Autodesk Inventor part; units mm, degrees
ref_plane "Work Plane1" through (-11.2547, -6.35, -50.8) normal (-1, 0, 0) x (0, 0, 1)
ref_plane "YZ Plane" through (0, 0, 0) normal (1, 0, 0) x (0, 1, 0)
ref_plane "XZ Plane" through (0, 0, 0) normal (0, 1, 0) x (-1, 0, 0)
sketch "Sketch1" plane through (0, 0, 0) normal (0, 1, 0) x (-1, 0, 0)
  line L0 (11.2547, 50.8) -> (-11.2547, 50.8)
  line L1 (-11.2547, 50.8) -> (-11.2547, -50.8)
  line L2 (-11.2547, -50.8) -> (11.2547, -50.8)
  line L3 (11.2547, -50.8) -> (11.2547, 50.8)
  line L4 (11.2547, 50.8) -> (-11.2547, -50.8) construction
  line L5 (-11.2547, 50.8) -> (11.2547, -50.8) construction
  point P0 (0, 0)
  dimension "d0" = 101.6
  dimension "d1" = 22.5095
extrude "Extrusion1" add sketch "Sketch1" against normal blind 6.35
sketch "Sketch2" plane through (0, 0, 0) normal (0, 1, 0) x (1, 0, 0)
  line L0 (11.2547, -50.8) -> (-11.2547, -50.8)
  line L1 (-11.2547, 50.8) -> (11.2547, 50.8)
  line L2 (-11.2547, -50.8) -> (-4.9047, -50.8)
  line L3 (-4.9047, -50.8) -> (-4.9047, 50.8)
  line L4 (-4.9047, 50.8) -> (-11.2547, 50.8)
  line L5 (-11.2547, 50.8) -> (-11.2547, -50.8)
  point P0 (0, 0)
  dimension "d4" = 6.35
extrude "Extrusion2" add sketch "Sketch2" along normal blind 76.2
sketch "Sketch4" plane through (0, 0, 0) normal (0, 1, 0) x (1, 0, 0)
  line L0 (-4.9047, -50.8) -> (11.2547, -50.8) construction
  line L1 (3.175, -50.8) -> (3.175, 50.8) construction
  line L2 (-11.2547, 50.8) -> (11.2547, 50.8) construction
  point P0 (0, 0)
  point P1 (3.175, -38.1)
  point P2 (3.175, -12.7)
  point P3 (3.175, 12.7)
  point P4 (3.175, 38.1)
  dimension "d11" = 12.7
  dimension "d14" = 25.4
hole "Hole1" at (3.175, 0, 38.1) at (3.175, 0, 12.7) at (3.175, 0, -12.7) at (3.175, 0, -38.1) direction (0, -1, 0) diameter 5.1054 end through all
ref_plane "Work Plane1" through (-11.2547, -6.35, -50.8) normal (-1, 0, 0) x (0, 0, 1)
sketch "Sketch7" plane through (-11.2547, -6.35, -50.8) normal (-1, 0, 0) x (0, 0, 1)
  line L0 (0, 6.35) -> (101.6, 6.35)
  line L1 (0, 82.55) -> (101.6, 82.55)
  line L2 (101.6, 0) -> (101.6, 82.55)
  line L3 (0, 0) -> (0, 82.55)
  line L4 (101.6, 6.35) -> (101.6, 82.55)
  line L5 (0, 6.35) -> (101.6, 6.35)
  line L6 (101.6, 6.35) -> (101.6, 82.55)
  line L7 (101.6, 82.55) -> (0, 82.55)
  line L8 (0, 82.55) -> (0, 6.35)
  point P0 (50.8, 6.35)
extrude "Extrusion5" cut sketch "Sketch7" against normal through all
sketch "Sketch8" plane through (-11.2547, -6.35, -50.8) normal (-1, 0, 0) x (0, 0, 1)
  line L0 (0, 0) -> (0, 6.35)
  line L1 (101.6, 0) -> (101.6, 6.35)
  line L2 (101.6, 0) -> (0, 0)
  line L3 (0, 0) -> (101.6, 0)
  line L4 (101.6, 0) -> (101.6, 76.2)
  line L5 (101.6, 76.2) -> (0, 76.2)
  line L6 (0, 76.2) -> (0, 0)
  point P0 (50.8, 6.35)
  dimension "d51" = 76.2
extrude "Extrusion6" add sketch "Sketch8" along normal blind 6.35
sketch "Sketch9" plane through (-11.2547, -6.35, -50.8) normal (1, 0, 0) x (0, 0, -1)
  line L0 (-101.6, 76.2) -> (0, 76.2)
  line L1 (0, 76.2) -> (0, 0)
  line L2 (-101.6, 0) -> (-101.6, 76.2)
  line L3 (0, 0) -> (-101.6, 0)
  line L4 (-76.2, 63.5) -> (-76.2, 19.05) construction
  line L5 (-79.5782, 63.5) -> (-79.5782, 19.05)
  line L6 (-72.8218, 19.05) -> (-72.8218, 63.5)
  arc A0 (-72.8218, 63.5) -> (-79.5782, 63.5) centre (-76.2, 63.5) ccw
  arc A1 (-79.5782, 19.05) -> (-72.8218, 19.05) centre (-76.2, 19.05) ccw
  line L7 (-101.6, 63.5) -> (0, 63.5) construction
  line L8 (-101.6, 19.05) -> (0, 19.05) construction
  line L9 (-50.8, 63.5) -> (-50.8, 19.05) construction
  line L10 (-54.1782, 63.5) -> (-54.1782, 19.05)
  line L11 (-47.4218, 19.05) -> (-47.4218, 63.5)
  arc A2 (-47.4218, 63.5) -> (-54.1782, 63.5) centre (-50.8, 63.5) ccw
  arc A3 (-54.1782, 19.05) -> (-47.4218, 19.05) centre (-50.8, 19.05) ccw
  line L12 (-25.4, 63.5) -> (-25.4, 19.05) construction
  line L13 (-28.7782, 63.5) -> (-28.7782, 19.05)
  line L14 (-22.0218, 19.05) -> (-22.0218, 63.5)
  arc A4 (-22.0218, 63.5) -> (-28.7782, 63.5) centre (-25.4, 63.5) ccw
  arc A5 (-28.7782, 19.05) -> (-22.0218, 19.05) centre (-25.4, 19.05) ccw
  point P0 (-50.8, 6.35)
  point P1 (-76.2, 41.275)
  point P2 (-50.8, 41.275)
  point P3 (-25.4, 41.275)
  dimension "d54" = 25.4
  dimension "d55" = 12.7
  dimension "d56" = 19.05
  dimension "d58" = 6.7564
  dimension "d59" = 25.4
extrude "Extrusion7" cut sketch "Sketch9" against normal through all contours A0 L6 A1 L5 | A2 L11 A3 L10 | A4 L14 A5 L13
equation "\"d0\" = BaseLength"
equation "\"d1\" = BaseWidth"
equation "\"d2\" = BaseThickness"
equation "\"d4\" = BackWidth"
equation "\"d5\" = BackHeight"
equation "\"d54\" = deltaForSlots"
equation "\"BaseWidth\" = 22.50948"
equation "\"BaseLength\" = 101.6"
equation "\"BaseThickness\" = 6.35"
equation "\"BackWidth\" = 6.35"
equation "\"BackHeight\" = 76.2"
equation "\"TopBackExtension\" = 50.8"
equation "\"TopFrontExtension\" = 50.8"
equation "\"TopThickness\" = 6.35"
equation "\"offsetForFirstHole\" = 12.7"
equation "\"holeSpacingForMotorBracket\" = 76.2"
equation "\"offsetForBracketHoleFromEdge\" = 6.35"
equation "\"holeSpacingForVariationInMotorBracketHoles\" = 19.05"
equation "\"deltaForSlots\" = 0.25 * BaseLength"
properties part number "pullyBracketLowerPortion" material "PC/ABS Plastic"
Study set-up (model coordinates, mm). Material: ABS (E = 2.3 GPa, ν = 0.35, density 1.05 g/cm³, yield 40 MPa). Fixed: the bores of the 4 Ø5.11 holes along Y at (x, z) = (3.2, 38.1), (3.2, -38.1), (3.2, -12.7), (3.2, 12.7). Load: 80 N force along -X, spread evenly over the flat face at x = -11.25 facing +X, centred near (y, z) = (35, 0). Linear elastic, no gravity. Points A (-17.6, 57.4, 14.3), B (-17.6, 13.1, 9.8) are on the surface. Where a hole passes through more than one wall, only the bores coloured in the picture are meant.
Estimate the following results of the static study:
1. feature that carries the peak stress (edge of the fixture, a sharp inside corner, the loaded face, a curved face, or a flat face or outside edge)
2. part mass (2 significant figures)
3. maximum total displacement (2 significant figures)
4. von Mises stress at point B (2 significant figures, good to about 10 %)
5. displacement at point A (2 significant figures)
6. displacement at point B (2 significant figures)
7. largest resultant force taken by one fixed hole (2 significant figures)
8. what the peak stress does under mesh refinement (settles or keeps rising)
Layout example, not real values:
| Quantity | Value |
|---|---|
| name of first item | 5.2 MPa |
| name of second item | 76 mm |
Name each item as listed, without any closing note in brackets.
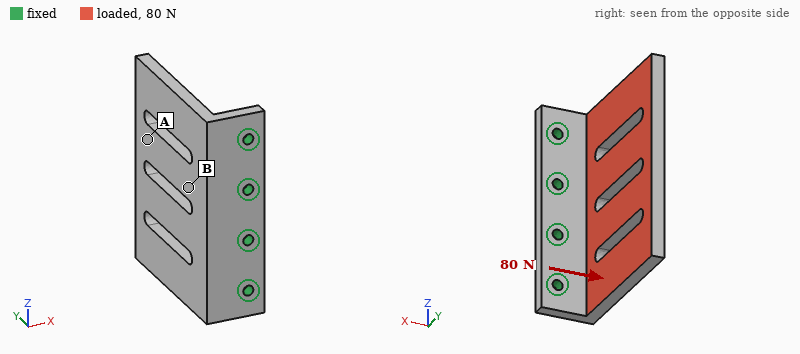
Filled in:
| Quantity | Value |
|---|---|
| feature that carries the peak stress | edge of the fixture |
| part mass | 60 g |
| maximum total displacement | 1.6 mm |
| von Mises stress at point B | 3.2 MPa |
| displacement at point A | 1.2 mm |
| displacement at point B | 0.26 mm |
| largest resultant force taken by one fixed hole | 22 N |
| what the peak stress does under mesh refinement | keeps rising |
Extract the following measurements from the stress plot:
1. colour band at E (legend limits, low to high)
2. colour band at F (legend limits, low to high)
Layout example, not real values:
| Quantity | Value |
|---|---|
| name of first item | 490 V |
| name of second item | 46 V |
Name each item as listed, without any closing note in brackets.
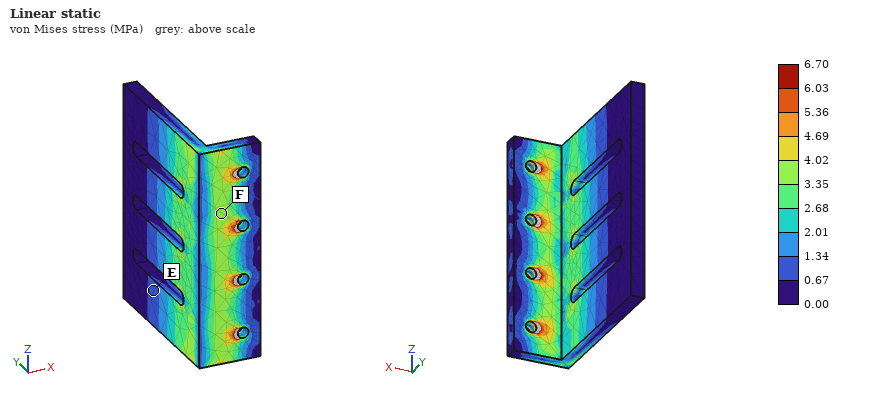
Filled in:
| Quantity | Value |
|---|---|
| colour band at E | 0.67 to 1.34 MPa |
| colour band at F | 3.35 to 4.02 MPa |
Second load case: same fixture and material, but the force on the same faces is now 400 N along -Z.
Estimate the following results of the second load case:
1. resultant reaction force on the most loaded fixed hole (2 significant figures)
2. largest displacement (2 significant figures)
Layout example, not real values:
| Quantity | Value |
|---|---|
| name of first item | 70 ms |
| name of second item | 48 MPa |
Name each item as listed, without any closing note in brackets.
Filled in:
| Quantity | Value |
|---|---|
| resultant reaction force on the most loaded fixed hole | 210 N |
| largest displacement | 0.98 mm |
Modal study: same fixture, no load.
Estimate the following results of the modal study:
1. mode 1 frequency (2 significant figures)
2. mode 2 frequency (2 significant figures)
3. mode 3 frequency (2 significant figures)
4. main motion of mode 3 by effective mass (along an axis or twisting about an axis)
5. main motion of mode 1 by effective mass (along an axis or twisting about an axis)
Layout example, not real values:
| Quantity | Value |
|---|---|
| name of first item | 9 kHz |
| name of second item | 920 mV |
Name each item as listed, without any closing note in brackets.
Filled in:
| Quantity | Value |
|---|---|
| mode 1 frequency | 220 Hz |
| mode 2 frequency | 420 Hz |
| mode 3 frequency | 790 Hz |
| main motion of mode 3 by effective mass | along Z |
| main motion of mode 1 by effective mass | along X |
